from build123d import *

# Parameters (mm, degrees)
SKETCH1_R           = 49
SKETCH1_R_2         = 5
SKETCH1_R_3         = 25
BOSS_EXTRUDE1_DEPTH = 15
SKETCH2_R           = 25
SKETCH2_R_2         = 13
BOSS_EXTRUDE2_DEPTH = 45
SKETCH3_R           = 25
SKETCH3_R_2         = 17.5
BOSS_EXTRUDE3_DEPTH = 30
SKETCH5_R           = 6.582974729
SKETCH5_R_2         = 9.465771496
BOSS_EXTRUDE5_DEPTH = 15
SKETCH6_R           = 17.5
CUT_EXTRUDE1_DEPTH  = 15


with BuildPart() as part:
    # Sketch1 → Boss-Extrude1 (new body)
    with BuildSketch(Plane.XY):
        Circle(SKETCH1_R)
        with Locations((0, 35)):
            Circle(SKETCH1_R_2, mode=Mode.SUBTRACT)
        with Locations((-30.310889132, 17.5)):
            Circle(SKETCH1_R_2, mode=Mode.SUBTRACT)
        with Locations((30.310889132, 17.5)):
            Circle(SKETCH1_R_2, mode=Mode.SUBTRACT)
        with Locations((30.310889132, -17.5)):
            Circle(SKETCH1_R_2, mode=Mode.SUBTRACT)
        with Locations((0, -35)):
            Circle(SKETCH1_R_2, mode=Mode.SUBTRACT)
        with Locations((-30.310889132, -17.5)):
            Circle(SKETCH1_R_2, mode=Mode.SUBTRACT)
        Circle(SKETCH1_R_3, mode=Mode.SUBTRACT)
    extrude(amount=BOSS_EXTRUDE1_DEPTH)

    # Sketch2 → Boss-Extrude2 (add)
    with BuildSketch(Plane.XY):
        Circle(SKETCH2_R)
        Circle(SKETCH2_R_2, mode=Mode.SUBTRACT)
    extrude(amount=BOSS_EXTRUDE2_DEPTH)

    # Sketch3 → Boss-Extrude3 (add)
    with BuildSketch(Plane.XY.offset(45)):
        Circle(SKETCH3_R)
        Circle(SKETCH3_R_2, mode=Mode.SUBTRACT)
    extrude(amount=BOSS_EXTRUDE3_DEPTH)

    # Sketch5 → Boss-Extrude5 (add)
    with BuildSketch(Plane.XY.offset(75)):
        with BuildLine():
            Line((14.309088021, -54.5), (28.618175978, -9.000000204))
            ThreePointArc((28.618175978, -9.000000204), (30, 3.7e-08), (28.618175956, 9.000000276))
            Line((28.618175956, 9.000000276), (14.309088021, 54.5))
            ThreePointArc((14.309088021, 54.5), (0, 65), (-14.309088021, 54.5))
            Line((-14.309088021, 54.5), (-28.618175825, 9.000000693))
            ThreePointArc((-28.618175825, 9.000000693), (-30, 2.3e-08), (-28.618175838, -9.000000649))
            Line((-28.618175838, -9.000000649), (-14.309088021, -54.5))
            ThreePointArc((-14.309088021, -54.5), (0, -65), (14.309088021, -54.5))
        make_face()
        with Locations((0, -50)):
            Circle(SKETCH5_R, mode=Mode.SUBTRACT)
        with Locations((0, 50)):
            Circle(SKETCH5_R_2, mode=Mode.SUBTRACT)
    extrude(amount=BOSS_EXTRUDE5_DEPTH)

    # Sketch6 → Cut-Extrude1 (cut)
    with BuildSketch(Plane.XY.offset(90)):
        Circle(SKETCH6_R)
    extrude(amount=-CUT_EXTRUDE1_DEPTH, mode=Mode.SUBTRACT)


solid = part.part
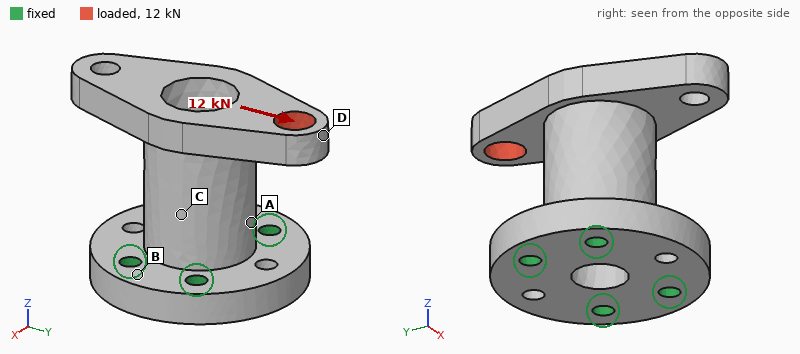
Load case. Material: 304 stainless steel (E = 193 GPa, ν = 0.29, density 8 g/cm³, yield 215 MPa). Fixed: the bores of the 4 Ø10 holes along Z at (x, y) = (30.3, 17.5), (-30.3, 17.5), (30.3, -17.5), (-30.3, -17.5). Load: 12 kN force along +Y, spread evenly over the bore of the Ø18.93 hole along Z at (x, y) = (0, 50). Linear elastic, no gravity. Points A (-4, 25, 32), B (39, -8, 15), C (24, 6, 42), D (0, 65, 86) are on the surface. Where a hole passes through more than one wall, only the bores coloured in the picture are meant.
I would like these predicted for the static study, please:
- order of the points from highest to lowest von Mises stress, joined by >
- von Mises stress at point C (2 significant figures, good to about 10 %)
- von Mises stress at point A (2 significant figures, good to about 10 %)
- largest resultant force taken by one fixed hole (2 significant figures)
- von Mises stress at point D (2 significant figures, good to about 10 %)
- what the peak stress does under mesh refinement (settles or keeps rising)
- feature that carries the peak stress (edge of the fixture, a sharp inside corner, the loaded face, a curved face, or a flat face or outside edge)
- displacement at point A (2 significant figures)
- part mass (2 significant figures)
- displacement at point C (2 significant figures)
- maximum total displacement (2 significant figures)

A > D > C > B
25 MPa
57 MPa
12 kN
42 MPa
keeps rising
edge of the fixture
0.025 mm
1.9 kg
0.026 mm
0.13 mm
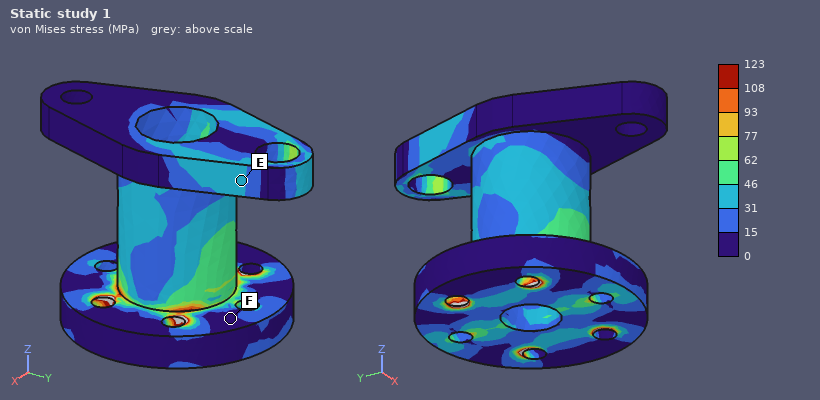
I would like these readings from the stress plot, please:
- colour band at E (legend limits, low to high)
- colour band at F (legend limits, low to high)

31 to 46 MPa
0 to 15 MPa
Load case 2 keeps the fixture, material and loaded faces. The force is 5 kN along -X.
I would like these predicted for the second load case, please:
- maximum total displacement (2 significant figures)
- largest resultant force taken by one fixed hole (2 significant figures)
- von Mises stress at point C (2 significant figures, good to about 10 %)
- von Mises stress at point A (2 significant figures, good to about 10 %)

74 µm
4.5 kN
30 MPa
28 MPa
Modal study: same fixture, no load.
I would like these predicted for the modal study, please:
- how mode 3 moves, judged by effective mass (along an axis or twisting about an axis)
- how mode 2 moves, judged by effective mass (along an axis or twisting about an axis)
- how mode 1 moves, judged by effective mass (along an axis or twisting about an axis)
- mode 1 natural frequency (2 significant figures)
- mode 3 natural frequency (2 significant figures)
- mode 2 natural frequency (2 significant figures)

twisting about Z
along X
along Y
2300 Hz
4200 Hz
2900 Hz
